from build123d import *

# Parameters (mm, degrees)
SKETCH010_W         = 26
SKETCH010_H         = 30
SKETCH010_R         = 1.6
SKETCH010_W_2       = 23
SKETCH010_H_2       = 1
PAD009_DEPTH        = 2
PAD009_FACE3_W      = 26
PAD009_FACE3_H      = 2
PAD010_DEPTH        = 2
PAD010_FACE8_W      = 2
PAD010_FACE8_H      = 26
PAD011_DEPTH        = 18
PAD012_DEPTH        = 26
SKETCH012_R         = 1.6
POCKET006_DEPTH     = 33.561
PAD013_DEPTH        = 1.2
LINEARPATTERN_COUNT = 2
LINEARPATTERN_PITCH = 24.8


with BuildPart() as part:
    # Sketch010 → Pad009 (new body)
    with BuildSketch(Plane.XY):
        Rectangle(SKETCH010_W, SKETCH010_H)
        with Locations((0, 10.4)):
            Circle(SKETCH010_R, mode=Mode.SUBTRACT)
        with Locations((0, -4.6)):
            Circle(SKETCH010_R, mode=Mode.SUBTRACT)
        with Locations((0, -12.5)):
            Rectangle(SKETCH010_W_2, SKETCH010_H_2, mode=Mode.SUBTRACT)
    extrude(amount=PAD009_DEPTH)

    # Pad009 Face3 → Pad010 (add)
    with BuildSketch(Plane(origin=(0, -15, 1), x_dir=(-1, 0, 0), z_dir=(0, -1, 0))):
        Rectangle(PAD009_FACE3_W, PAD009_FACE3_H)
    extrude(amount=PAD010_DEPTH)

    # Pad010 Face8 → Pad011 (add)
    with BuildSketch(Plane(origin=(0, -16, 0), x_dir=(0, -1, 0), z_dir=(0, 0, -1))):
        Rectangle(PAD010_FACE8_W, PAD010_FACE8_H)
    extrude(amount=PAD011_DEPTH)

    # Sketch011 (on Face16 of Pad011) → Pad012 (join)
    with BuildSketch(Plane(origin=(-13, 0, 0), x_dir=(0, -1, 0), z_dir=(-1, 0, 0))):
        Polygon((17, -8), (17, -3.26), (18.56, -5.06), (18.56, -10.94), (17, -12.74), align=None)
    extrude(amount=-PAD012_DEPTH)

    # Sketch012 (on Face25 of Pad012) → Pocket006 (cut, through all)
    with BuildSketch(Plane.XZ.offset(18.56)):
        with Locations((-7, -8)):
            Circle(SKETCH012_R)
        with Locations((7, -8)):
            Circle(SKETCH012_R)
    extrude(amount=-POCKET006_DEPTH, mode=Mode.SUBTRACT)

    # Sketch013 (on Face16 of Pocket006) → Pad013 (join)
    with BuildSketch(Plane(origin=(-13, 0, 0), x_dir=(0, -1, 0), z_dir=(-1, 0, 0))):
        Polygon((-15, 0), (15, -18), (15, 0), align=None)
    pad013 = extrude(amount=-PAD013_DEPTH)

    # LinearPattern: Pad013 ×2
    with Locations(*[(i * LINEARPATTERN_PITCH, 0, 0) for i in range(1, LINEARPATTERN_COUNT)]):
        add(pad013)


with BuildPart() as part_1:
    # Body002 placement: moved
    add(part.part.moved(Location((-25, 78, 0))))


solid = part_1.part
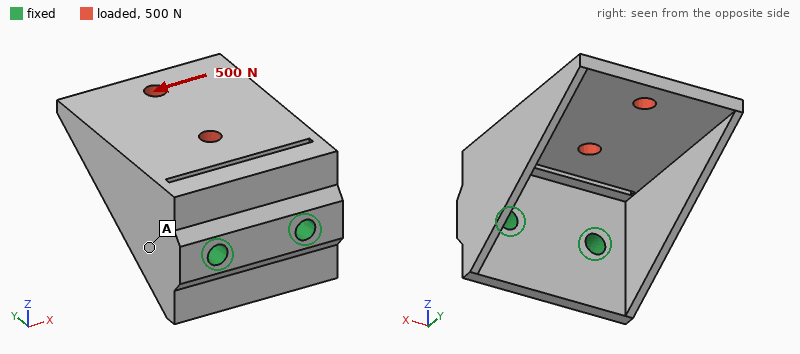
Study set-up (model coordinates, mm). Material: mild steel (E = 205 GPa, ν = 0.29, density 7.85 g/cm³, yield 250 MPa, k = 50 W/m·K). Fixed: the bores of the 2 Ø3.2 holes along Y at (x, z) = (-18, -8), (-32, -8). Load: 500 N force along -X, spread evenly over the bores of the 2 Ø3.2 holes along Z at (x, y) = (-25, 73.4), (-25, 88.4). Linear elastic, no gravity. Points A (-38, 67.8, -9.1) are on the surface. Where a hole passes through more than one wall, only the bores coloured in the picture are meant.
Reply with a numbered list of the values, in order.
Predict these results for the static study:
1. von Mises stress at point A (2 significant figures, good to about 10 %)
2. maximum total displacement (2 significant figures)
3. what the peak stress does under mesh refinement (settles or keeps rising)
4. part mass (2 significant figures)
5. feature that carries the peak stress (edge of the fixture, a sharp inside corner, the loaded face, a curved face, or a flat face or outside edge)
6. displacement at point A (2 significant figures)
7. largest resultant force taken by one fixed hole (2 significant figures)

1. 28 MPa
2. 64 µm
3. keeps rising
4. 27 g
5. a sharp inside corner
6. 11 µm
7. 570 N
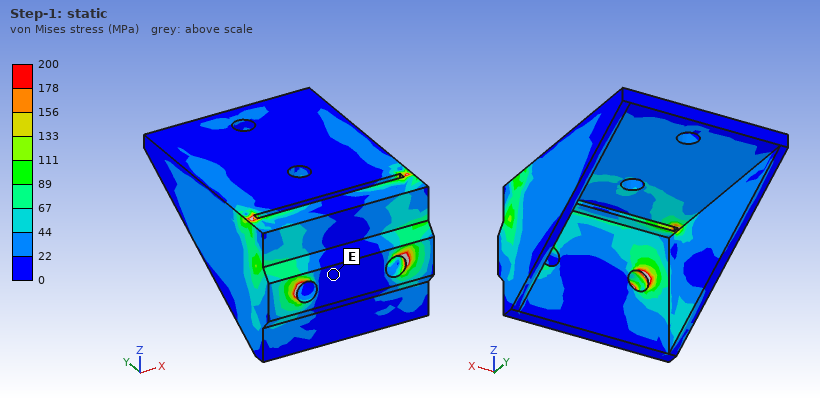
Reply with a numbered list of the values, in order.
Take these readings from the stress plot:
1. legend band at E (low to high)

1. 0 to 22 MPa
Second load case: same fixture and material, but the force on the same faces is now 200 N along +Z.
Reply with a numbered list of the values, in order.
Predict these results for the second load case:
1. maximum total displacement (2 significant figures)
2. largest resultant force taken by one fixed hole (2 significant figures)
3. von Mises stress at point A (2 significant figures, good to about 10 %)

1. 54 µm
2. 100 N
3. 16 MPa
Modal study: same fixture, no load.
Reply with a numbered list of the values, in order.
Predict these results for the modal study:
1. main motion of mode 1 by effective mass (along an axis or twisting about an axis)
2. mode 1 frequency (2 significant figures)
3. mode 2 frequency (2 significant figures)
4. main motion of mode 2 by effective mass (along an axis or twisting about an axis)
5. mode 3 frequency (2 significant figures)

1. along Z
2. 3900 Hz
3. 4400 Hz
4. along X
5. 10 kHz
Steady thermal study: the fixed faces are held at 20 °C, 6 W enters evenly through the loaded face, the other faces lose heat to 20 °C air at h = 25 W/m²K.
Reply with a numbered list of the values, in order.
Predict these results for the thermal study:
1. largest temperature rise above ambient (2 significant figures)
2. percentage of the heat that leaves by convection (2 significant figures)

1. 51 K
2. 34 %
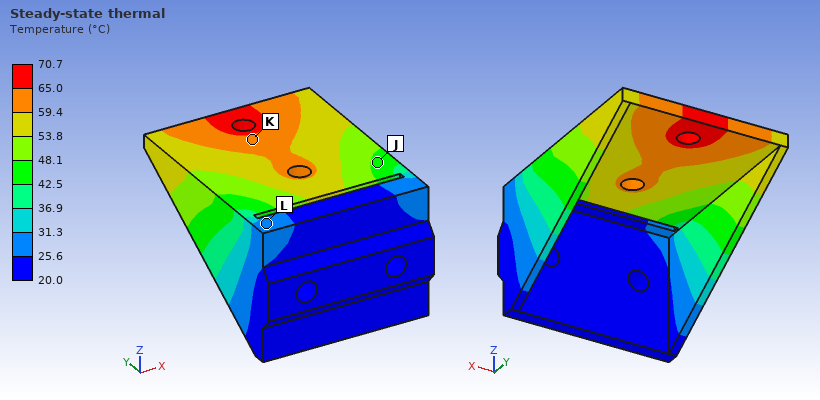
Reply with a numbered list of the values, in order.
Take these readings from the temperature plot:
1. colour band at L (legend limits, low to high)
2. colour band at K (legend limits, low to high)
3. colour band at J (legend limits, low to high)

1. 25.6 to 31.3 °C
2. 59.4 to 65.0 °C
3. 42.5 to 48.1 °C
